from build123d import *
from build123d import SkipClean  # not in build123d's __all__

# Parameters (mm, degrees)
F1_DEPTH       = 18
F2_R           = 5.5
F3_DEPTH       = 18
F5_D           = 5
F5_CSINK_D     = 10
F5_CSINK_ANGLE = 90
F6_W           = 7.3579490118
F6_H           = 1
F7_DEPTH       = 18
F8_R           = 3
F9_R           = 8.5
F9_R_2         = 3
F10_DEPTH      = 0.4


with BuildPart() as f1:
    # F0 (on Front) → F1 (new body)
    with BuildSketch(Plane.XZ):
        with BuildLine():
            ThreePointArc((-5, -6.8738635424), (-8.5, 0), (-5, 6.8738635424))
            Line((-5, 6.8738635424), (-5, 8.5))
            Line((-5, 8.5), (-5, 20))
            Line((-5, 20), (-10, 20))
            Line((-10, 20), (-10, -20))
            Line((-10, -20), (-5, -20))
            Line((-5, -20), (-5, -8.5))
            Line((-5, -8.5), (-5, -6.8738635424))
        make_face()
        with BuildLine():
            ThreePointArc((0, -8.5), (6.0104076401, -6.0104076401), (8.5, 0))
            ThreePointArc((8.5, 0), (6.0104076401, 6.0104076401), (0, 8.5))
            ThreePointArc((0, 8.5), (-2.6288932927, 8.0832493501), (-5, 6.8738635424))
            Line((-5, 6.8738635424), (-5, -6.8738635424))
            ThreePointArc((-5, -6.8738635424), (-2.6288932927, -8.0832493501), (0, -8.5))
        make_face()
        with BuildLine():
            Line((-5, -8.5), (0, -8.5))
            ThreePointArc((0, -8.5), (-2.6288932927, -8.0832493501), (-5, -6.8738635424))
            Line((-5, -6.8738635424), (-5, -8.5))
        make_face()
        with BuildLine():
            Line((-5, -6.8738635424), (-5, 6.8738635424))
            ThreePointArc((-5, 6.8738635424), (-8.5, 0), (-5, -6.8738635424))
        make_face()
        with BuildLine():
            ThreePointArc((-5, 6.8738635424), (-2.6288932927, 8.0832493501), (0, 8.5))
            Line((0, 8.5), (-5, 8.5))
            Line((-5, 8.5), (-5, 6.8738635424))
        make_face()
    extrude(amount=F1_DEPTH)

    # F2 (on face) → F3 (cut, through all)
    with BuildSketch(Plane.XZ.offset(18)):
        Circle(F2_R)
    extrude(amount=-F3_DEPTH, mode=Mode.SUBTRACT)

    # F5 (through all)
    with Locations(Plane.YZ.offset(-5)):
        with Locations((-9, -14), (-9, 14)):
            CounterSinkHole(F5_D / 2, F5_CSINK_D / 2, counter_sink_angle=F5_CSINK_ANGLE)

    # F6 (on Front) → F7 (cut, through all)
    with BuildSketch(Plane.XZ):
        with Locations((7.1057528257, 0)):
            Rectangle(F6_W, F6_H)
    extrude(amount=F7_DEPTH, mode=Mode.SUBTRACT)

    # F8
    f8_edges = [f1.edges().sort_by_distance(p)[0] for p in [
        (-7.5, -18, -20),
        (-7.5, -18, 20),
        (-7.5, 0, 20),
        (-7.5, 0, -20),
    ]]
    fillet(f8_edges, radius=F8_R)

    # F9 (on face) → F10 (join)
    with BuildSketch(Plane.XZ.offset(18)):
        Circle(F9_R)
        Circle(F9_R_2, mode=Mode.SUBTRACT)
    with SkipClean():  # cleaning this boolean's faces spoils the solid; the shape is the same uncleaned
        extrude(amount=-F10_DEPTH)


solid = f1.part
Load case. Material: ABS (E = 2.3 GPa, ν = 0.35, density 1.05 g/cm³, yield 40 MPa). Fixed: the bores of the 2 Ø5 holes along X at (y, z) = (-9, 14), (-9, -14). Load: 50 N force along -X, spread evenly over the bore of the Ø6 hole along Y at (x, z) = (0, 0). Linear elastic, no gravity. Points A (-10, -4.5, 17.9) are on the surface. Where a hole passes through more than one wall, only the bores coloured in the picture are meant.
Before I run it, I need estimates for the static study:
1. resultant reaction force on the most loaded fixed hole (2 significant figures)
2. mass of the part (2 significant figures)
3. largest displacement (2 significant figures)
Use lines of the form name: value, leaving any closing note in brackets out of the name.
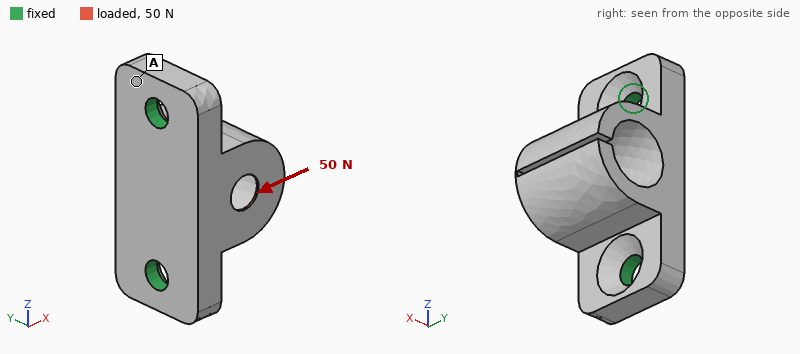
resultant reaction force on the most loaded fixed hole: 31 N
mass of the part: 5.3 g
largest displacement: 85 µm
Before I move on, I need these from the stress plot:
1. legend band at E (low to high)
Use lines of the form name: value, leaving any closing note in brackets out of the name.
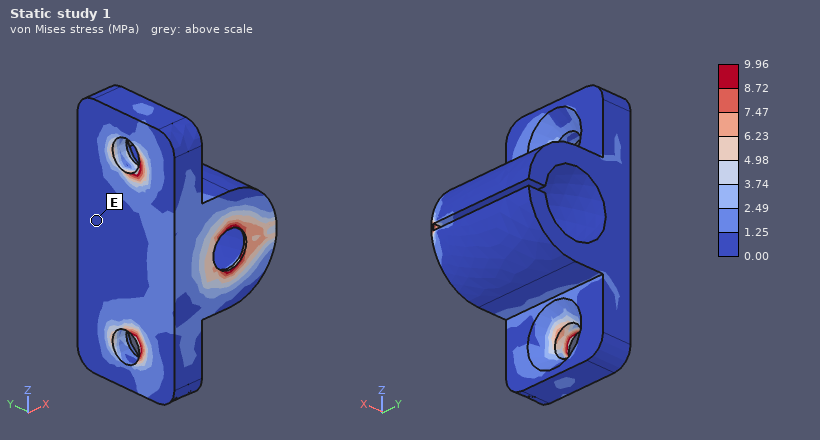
legend band at E: 0.00 to 1.25 MPa
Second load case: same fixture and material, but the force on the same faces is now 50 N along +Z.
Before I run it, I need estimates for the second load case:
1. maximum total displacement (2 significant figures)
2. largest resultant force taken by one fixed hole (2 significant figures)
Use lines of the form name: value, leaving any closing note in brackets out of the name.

maximum total displacement: 47 µm
largest resultant force taken by one fixed hole: 34 N
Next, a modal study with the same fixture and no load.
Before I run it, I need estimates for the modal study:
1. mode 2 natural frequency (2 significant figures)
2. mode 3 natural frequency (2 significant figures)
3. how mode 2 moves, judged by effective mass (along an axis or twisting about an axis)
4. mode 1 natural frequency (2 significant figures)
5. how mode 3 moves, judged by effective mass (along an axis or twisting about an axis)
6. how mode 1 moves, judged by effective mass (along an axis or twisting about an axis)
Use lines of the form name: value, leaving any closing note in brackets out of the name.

mode 2 natural frequency: 3900 Hz
mode 3 natural frequency: 4400 Hz
how mode 2 moves, judged by effective mass: along X
mode 1 natural frequency: 2900 Hz
how mode 3 moves, judged by effective mass: along Z
how mode 1 moves, judged by effective mass: along Y
